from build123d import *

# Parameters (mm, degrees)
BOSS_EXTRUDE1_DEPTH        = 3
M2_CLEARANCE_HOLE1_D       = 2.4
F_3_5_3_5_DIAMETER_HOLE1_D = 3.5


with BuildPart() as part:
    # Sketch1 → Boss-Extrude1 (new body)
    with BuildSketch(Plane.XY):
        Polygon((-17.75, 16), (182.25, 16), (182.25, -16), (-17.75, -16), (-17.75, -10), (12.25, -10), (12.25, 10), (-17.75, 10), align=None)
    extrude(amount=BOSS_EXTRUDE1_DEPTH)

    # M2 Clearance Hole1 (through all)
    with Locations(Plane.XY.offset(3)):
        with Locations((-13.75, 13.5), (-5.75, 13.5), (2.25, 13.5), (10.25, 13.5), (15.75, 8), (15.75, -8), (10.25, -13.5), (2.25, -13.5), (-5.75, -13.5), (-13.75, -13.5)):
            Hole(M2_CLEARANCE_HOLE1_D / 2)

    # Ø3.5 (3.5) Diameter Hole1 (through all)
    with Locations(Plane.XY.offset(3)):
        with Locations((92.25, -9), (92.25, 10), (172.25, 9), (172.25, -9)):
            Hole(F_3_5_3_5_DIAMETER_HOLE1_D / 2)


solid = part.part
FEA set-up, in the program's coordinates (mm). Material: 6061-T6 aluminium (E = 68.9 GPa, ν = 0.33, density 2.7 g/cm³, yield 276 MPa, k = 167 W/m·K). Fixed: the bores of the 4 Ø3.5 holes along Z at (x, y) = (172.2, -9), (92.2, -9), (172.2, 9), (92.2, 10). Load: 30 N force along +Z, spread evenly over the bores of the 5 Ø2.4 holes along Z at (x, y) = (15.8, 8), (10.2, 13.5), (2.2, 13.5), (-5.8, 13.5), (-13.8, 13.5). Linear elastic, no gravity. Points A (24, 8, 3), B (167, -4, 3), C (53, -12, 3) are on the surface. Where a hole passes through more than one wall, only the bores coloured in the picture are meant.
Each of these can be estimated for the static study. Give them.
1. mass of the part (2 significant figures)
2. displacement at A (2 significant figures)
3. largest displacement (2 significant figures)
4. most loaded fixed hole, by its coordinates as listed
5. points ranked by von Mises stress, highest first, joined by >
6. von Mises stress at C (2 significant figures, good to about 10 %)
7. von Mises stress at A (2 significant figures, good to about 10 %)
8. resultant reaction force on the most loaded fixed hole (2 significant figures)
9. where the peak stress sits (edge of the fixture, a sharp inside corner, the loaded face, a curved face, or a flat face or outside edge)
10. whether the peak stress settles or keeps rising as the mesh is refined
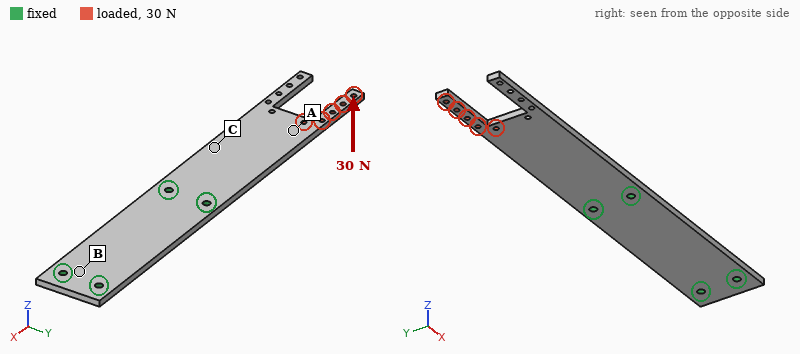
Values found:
46 g
0.96 mm
2.2 mm
(92.2, 10)
C > A > B
32 MPa
21 MPa
31 N
edge of the fixture
keeps rising
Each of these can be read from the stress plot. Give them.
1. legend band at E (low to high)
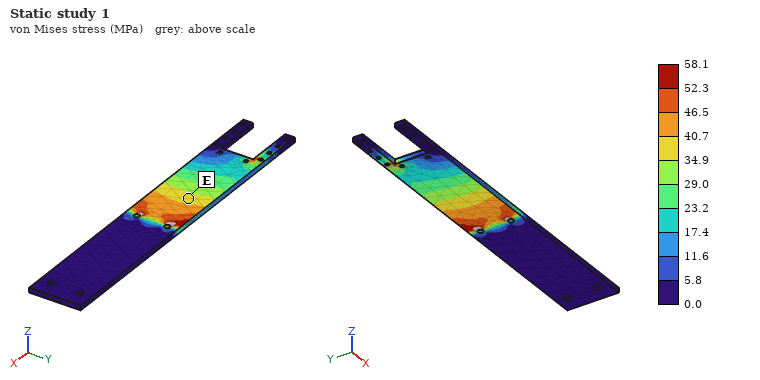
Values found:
34.9 to 40.7 MPa
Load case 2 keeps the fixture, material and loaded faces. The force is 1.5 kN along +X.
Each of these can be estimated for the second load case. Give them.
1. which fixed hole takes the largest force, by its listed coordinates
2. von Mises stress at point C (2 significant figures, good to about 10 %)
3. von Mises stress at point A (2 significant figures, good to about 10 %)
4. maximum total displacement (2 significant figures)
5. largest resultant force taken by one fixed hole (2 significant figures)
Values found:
(92.2, 10)
12 MPa
32 MPa
0.31 mm
1.5 kN
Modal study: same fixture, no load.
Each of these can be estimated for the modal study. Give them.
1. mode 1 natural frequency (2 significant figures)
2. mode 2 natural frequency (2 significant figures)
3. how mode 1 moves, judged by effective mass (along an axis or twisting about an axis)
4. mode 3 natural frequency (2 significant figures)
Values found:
290 Hz
1300 Hz
along Z
1400 Hz
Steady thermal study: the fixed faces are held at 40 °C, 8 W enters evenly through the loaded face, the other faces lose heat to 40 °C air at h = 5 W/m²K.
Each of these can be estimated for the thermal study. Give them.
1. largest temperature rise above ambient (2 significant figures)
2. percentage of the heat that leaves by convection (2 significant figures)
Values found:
85 K
10 %
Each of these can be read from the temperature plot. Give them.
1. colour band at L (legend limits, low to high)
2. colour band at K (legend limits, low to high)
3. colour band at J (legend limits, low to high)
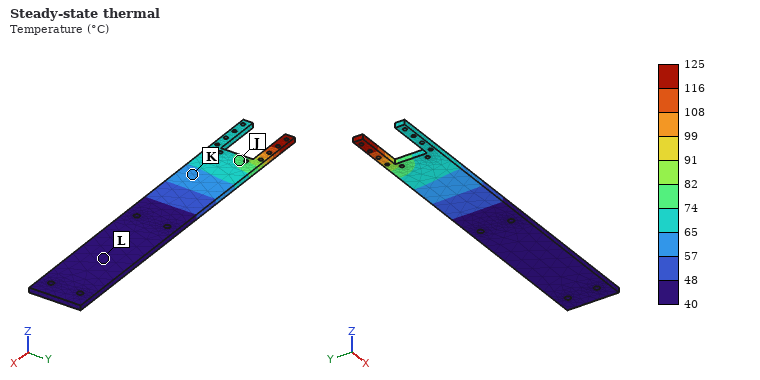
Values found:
40 to 48 °C
57 to 65 °C
74 to 82 °C
